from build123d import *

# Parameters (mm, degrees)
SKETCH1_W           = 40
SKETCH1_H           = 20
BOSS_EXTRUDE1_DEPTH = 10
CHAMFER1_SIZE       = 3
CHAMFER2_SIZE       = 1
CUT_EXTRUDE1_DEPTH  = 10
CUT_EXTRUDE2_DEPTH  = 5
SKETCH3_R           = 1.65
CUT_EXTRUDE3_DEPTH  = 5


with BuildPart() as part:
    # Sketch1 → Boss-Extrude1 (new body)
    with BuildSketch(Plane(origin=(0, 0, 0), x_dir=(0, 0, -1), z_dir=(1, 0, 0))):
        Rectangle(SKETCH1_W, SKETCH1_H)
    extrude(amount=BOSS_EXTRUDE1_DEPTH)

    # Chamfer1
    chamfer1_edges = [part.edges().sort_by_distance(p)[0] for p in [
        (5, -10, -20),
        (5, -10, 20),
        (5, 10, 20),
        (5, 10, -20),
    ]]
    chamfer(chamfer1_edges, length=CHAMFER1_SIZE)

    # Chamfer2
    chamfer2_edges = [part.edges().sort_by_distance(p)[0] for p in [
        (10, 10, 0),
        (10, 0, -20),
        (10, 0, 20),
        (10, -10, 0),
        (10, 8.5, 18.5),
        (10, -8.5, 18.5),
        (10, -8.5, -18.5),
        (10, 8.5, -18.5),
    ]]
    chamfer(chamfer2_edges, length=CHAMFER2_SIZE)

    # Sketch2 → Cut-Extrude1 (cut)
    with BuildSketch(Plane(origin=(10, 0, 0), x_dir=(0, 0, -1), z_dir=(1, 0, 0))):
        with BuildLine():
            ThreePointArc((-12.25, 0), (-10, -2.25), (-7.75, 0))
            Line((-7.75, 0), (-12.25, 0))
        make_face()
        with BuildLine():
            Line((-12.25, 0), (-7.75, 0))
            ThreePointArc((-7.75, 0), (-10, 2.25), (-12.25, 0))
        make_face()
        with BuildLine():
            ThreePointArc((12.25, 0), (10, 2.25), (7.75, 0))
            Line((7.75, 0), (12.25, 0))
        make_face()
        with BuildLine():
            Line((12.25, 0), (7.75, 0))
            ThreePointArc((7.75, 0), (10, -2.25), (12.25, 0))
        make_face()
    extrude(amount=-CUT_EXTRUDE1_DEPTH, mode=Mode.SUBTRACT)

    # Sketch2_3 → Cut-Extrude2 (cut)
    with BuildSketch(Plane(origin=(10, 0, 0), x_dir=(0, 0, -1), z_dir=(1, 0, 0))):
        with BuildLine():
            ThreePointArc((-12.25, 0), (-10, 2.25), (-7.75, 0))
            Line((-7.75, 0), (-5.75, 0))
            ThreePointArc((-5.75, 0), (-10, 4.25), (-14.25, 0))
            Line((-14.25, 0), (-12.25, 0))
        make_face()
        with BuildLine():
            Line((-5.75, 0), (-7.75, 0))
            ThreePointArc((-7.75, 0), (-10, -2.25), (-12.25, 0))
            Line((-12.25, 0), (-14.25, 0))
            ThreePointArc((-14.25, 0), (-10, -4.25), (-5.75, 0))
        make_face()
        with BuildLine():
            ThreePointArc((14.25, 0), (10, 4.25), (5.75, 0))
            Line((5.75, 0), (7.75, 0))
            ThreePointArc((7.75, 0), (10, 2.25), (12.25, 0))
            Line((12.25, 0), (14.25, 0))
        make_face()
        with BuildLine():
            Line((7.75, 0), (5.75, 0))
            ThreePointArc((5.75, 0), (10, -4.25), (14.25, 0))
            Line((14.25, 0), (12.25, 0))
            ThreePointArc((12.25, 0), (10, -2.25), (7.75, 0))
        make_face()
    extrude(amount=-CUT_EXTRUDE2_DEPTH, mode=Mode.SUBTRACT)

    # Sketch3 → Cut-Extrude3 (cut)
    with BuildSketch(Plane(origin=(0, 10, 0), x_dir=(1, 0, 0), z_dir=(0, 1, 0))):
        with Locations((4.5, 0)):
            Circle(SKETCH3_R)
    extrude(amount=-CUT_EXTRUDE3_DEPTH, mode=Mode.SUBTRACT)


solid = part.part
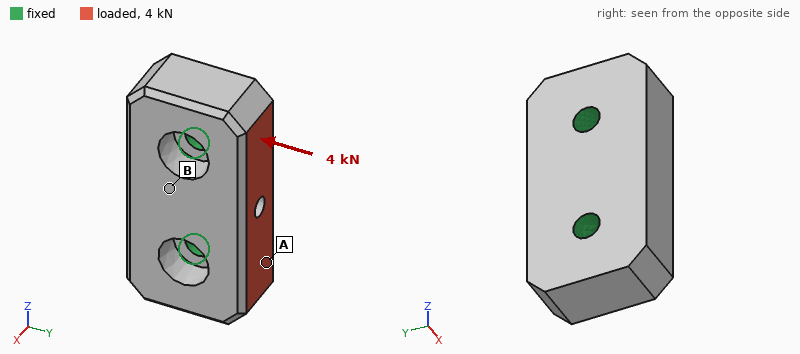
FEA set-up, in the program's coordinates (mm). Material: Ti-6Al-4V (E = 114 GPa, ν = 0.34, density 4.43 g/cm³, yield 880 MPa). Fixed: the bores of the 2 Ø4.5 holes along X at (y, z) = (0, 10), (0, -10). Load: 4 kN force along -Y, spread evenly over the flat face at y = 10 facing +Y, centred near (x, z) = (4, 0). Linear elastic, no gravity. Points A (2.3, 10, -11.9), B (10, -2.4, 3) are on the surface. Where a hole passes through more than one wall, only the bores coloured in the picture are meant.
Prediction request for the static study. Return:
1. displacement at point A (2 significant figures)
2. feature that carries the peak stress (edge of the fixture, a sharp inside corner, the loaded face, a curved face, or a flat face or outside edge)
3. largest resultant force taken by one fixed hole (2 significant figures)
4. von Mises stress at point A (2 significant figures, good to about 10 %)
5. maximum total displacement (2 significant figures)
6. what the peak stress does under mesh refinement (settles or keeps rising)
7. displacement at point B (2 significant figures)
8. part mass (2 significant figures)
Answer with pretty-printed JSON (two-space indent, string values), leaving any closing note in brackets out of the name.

{
  "displacement at point A": "3.8 µm",
  "feature that carries the peak stress": "edge of the fixture",
  "largest resultant force taken by one fixed hole": "2.0 kN",
  "von Mises stress at point A": "16 MPa",
  "maximum total displacement": "5.9 µm",
  "what the peak stress does under mesh refinement": "keeps rising",
  "displacement at point B": "3.9 µm",
  "part mass": "31 g"
}
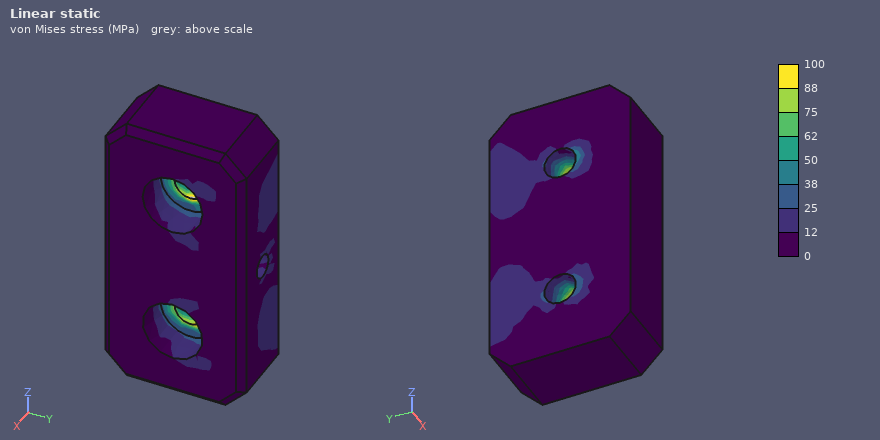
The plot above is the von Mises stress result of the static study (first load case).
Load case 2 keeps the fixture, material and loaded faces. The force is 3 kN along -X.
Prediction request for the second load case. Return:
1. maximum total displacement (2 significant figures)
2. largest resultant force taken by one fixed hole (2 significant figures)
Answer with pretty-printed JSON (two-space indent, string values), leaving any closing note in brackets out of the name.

{
  "maximum total displacement": "20 µm",
  "largest resultant force taken by one fixed hole": "1.5 kN"
}
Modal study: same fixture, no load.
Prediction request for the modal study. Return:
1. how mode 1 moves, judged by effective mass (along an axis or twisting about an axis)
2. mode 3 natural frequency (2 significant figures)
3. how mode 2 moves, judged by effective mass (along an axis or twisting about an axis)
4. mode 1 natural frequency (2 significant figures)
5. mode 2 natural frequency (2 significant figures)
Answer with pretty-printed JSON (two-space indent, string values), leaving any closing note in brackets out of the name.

{
  "how mode 1 moves, judged by effective mass": "along Y",
  "mode 3 natural frequency": "31 kHz",
  "how mode 2 moves, judged by effective mass": "twisting about X",
  "mode 1 natural frequency": "20 kHz",
  "mode 2 natural frequency": "30 kHz"
}
